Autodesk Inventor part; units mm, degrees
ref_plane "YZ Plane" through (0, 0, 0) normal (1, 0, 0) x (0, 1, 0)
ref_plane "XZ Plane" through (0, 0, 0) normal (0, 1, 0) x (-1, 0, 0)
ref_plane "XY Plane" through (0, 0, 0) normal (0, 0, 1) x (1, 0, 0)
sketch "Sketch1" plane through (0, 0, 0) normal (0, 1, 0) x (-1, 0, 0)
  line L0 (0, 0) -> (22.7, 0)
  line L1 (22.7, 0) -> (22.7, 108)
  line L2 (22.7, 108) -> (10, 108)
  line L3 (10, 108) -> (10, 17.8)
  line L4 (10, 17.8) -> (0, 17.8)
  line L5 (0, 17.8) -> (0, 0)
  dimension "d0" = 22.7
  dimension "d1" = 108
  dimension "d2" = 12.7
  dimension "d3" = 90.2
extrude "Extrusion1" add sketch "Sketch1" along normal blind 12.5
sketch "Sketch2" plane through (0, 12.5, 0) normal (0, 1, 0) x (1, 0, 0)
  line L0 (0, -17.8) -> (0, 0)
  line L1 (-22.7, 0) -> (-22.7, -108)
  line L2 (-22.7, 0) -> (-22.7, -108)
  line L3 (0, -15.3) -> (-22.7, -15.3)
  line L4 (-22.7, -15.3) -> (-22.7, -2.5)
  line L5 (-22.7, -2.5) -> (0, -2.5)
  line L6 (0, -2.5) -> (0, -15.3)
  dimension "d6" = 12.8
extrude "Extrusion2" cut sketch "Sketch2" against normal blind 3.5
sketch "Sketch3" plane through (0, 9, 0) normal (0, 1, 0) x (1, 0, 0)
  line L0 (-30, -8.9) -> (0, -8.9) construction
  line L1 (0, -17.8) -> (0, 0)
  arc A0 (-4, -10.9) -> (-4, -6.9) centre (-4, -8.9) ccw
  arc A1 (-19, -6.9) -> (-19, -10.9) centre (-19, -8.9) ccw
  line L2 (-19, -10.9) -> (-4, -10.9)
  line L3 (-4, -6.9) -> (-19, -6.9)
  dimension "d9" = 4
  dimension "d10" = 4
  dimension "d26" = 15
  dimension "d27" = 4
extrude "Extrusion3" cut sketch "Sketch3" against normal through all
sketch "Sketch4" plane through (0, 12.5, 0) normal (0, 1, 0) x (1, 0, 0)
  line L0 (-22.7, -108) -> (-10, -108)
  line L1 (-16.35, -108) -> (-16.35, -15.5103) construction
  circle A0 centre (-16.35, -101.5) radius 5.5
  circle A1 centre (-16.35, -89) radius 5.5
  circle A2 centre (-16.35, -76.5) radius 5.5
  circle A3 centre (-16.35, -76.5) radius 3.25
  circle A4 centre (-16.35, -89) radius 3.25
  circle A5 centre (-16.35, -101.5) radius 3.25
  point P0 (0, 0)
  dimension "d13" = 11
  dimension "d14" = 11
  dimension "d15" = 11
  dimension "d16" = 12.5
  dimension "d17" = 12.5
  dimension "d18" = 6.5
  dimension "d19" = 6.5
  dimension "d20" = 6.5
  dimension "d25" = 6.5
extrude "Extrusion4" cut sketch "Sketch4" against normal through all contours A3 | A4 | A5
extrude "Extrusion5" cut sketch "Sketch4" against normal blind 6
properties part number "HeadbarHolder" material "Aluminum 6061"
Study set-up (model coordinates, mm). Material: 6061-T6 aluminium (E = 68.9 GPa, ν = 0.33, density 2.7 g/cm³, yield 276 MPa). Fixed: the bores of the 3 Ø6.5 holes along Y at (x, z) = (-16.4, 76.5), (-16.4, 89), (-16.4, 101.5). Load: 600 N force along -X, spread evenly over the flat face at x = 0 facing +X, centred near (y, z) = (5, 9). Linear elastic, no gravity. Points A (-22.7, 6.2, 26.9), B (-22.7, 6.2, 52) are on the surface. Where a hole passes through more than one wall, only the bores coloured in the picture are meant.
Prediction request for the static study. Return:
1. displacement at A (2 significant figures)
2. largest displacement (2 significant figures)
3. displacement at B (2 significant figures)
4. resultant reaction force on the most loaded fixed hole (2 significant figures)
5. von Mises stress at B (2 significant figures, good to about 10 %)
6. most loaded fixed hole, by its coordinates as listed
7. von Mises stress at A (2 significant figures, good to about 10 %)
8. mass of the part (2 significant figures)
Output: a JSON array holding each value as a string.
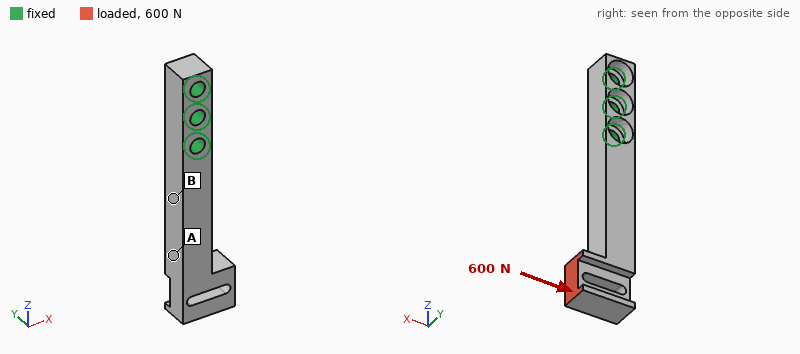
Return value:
["0.34 mm", "0.66 mm", "0.12 mm", "1.4 kN", "77 MPa", "(-16.4, 76.5)", "33 MPa", "41 g"]
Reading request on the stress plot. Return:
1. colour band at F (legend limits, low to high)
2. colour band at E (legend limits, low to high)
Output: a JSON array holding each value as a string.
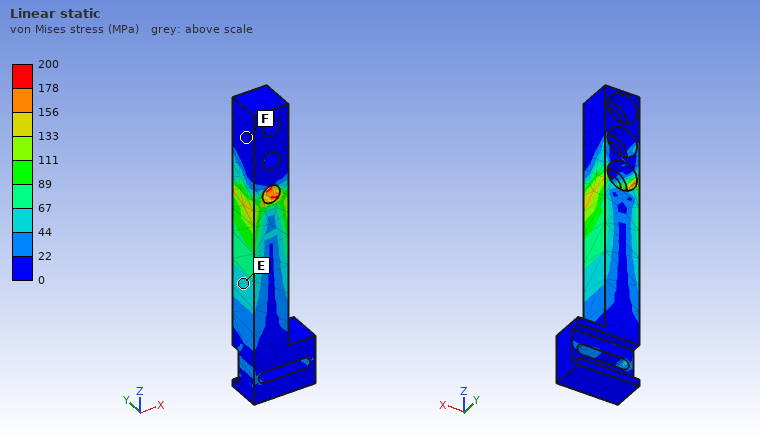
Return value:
["0 to 22 MPa", "44 to 67 MPa"]
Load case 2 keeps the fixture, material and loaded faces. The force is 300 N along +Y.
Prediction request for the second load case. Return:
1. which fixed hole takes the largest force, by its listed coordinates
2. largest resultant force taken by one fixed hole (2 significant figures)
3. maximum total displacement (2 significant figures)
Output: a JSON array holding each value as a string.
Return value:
["(-16.4, 76.5)", "900 N", "0.47 mm"]
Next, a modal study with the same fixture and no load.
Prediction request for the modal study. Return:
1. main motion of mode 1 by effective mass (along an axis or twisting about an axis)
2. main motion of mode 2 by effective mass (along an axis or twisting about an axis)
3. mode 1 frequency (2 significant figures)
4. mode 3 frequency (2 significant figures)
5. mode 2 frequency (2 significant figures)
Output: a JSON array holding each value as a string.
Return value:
["along Y", "along X", "1300 Hz", "6100 Hz", "1500 Hz"]
